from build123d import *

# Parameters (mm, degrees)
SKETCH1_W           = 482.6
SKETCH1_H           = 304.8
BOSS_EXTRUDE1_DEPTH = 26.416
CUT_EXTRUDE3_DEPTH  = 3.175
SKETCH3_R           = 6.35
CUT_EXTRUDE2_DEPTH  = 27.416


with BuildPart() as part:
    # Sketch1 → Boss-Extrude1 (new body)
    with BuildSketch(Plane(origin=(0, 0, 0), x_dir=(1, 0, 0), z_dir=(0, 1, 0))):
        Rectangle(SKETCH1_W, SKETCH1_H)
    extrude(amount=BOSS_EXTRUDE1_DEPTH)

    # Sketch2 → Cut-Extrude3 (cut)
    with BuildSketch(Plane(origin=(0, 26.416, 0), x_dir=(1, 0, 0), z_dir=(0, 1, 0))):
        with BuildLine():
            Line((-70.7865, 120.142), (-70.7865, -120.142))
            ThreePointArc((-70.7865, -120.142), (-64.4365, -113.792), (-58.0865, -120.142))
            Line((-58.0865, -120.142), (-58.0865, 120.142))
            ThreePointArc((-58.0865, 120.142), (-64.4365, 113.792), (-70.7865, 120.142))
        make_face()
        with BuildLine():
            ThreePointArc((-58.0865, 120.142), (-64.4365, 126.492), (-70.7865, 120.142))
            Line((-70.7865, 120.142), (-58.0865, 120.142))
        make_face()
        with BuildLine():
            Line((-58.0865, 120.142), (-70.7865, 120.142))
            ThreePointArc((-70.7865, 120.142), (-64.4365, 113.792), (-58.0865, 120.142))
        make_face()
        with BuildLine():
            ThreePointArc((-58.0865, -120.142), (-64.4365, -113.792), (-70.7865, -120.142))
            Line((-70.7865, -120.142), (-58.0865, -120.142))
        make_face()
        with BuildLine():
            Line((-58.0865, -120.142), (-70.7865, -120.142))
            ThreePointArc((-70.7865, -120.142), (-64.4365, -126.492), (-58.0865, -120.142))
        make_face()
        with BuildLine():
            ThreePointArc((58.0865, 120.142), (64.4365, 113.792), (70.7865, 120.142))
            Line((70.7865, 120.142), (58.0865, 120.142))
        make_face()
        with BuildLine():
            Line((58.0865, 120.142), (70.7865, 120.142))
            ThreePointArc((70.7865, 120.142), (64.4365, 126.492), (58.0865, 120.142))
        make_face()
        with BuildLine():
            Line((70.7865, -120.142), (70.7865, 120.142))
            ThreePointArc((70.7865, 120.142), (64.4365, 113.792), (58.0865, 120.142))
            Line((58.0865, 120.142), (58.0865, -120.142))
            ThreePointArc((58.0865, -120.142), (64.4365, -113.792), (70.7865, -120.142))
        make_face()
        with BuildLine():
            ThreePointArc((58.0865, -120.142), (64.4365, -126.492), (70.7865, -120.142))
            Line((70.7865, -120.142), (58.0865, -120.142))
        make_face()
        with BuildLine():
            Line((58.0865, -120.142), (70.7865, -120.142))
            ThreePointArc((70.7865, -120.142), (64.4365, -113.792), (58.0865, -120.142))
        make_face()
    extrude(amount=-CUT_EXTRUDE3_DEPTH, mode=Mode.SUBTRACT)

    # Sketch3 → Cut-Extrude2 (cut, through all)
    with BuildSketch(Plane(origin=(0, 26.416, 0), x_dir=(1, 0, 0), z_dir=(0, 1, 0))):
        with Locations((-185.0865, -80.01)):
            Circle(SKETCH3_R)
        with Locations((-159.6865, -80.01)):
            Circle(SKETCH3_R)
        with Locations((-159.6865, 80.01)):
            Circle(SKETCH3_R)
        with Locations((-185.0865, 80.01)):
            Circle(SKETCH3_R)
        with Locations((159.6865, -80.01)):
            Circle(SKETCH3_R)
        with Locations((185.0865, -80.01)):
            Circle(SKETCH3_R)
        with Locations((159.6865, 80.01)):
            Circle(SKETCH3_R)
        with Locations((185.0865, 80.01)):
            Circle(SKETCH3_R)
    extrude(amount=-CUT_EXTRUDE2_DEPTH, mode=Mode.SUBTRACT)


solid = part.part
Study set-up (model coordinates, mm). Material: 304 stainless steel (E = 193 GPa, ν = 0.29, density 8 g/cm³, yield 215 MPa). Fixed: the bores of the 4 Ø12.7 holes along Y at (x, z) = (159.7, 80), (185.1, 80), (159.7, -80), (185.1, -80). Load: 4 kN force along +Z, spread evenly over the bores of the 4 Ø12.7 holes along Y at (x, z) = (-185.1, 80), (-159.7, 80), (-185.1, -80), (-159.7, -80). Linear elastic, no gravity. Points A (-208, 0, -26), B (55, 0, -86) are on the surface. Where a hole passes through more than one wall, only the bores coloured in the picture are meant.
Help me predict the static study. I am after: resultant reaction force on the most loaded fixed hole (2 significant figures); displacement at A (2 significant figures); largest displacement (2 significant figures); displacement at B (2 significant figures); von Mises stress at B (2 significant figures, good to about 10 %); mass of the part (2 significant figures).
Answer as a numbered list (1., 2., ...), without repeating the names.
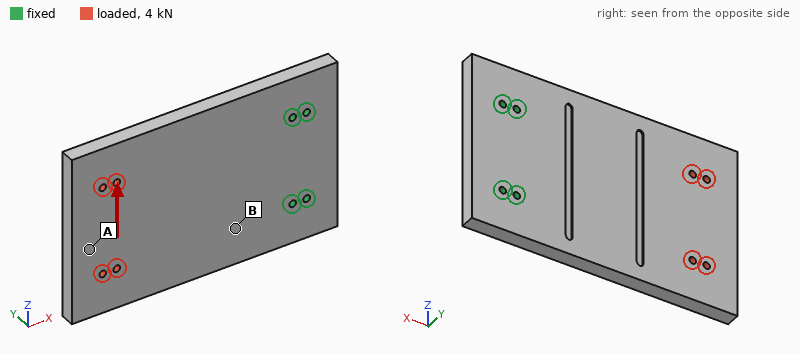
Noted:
1. 5.6 kN
2. 11 µm
3. 13 µm
4. 3.0 µm
5. 1.6 MPa
6. 31 kg
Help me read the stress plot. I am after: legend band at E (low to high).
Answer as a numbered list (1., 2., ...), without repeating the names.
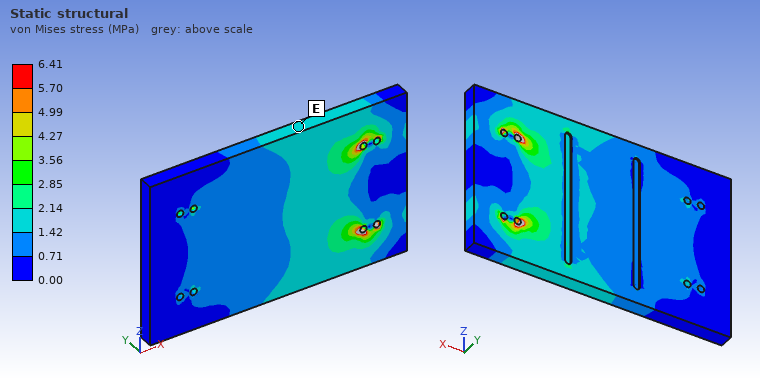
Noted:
1. 1.42 to 2.14 MPa
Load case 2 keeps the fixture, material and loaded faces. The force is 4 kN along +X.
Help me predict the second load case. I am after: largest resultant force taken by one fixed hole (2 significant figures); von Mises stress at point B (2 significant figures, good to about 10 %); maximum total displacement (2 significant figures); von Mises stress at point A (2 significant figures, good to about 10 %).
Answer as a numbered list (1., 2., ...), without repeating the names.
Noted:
1. 1.3 kN
2. 0.50 MPa
3. 1.4 µm
4. 0.24 MPa
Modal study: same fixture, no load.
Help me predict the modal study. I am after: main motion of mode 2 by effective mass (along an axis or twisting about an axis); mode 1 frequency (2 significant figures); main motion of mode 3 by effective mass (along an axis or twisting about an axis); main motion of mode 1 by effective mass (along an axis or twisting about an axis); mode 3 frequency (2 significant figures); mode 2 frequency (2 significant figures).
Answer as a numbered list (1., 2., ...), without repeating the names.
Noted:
1. twisting about X
2. 120 Hz
3. along Y
4. along Y
5. 740 Hz
6. 370 Hz
